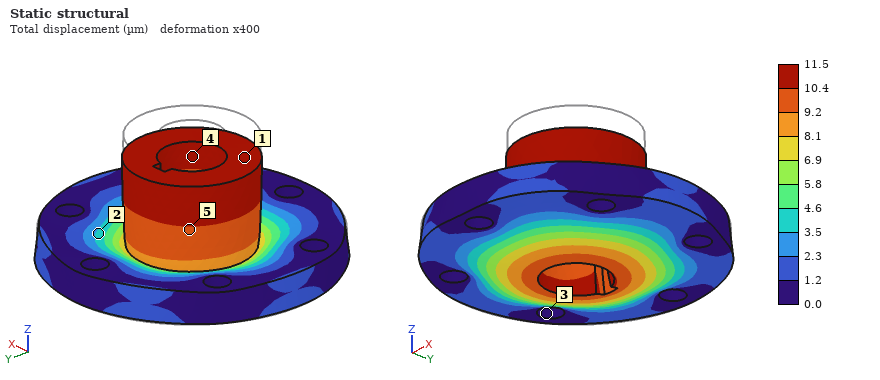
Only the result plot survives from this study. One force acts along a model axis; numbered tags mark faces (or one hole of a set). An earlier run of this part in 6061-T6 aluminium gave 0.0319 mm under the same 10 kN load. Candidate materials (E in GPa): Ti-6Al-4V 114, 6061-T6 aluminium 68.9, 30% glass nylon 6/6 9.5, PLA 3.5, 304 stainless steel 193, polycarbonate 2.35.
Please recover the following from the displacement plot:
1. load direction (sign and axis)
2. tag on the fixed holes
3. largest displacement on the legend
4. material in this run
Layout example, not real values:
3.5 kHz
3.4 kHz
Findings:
-Z
3
11.5 µm
304 stainless steel
